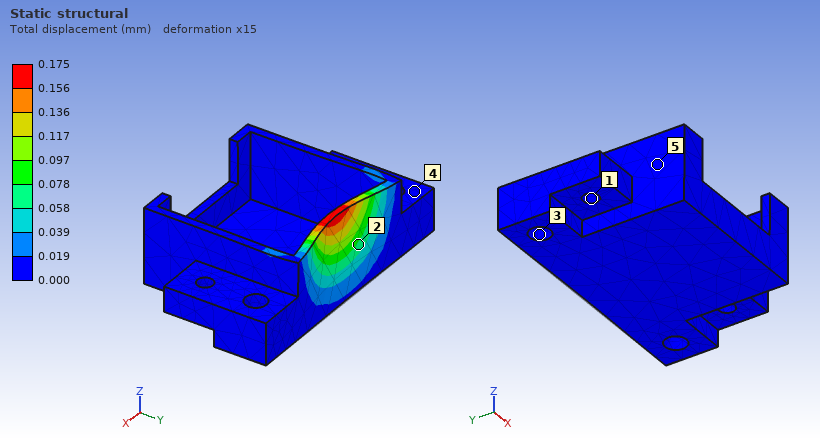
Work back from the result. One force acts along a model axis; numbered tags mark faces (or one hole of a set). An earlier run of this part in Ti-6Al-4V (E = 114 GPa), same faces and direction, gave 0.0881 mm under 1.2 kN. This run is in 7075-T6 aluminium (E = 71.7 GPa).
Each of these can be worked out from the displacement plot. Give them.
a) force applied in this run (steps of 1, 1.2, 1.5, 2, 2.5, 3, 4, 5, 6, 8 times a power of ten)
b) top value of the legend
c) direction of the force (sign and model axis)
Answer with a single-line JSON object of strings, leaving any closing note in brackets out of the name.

{"force applied in this run": "1.5 kN", "top value of the legend": "0.175 mm", "direction of the force": "-Y"}
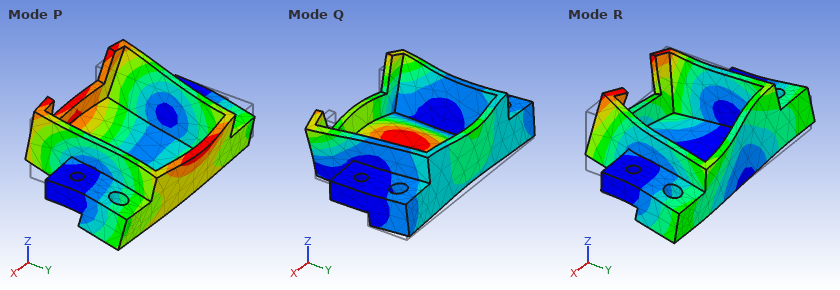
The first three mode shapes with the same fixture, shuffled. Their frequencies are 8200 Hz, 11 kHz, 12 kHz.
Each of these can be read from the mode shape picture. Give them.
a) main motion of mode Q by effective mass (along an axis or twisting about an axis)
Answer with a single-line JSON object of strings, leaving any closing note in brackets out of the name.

{"main motion of mode Q by effective mass": "along Z"}
